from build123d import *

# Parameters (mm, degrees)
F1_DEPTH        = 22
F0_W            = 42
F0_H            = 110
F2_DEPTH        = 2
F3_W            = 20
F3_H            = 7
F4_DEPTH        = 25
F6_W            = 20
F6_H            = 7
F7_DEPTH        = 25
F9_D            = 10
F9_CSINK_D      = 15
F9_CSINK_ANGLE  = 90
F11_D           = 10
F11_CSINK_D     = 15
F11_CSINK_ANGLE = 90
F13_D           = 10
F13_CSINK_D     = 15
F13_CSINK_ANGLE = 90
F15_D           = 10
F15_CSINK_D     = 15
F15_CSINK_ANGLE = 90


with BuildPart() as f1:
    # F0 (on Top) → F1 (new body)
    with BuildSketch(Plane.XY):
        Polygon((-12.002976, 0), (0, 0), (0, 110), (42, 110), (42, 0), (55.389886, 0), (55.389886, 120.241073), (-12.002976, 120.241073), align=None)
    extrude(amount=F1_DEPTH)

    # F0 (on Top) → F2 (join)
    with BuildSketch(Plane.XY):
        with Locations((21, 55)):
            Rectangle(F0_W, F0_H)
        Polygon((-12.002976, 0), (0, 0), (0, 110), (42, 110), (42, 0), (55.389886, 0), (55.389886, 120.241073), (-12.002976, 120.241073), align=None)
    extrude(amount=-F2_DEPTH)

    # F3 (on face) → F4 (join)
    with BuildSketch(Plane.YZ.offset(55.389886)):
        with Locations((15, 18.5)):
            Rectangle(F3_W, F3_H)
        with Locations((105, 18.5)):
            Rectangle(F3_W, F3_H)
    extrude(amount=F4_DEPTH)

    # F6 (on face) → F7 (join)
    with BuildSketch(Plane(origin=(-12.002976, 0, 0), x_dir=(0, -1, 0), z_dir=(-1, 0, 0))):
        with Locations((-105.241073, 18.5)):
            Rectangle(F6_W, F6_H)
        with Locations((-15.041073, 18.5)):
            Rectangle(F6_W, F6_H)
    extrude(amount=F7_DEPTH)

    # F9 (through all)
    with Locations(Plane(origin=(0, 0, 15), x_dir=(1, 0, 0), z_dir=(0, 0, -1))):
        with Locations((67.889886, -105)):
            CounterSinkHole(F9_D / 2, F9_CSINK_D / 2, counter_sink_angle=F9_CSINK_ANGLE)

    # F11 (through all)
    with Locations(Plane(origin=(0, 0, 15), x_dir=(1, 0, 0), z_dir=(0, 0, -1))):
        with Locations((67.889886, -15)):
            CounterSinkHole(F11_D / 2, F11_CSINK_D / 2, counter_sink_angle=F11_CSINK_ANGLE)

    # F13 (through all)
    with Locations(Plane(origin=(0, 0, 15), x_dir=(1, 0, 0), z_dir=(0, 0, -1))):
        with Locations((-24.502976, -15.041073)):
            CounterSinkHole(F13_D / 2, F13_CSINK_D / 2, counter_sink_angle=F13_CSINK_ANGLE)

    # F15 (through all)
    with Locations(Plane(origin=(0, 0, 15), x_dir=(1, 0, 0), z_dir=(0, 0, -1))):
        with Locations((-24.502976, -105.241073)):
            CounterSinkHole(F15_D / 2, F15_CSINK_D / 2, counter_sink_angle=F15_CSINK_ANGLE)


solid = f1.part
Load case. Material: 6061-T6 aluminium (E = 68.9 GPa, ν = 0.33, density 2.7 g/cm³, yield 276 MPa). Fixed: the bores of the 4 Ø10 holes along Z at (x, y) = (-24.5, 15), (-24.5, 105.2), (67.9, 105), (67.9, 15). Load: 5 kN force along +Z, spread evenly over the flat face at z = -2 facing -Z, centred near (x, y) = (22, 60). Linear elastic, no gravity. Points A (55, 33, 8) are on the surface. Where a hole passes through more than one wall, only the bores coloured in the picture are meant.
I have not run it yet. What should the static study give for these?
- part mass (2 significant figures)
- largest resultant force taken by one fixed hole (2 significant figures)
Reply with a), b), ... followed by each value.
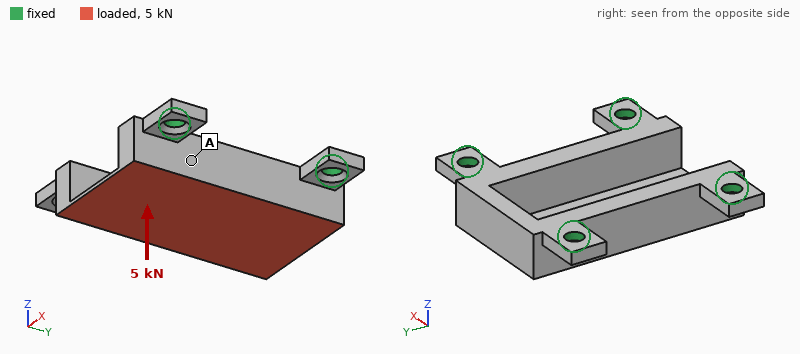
a) 280 g
b) 1.8 kN
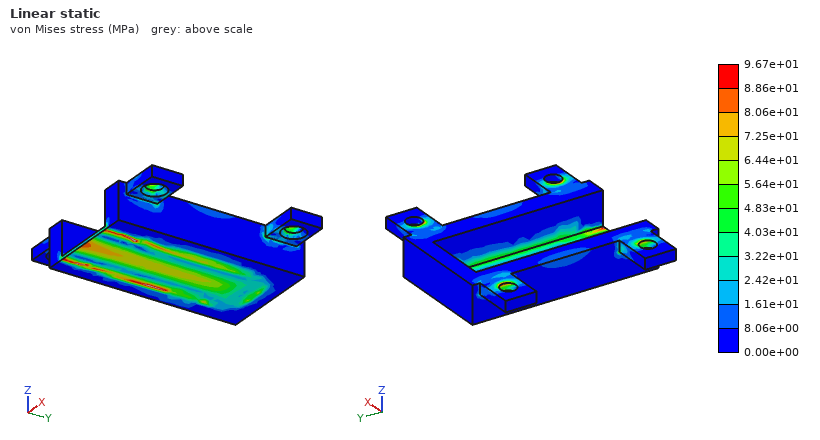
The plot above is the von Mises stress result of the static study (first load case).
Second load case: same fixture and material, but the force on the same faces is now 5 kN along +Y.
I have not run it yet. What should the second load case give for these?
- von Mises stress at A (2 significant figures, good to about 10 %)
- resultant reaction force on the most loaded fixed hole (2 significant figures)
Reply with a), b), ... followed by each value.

a) 7.3 MPa
b) 1.5 kN
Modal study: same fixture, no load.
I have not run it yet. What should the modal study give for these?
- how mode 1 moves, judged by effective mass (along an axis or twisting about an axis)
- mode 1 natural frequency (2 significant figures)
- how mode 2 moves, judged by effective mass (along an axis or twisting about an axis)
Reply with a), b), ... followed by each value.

a) along X
b) 3300 Hz
c) along Z
